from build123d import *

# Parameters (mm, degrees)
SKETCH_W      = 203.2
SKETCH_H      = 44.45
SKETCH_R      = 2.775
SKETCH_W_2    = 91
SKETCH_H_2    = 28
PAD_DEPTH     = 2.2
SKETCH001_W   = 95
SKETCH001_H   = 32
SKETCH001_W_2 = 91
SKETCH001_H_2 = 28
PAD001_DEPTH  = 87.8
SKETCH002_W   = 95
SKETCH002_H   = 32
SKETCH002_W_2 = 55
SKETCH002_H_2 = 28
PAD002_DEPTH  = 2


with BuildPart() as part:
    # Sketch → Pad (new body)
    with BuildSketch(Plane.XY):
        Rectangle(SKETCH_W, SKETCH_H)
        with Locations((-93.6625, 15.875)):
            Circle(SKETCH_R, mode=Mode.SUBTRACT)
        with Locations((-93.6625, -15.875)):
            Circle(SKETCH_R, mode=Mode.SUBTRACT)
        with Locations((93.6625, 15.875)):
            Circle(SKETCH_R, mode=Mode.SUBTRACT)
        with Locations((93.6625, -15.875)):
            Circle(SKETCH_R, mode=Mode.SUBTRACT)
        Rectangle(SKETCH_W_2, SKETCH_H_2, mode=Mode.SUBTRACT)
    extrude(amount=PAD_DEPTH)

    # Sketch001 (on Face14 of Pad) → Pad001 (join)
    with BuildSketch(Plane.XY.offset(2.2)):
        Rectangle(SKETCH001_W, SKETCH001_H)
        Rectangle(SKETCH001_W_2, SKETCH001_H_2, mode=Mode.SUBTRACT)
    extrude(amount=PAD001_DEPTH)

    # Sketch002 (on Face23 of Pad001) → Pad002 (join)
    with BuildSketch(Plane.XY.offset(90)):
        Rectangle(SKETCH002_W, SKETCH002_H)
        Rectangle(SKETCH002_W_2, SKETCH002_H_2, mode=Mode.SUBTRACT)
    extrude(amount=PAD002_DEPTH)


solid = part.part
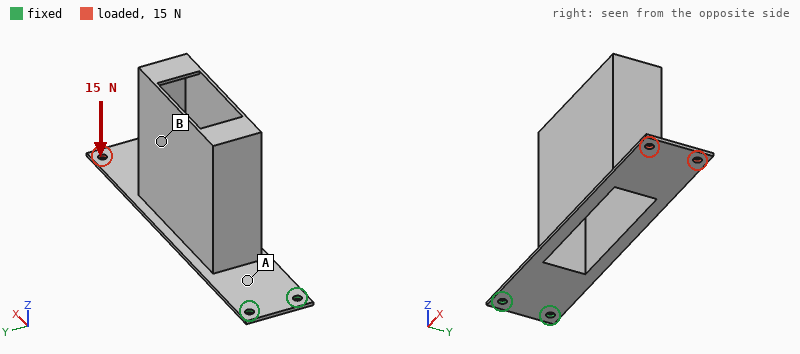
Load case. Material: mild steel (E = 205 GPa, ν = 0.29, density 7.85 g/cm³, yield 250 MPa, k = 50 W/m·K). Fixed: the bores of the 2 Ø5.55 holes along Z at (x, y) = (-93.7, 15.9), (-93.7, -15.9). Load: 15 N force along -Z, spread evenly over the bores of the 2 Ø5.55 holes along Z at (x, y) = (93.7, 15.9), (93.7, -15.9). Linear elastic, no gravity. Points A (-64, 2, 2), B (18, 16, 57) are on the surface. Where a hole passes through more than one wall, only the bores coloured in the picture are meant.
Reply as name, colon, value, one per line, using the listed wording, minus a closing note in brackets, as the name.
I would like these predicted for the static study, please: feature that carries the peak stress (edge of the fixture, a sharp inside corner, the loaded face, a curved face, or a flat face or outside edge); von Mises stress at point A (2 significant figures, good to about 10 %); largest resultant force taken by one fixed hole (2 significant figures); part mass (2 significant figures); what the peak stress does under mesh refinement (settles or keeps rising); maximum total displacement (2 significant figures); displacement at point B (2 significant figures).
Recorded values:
feature that carries the peak stress: edge of the fixture
von Mises stress at point A: 61 MPa
largest resultant force taken by one fixed hole: 7.7 N
part mass: 470 g
what the peak stress does under mesh refinement: keeps rising
maximum total displacement: 2.5 mm
displacement at point B: 1.5 mm
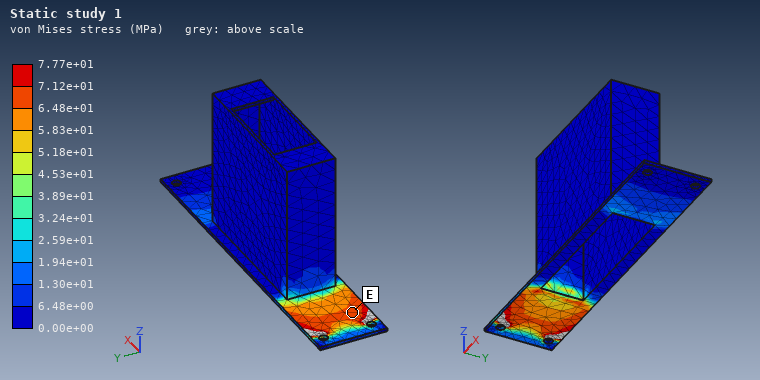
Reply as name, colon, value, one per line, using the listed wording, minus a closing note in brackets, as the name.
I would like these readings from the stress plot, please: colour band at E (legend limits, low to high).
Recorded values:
colour band at E: 6.48e+01 to 7.12e+01 MPa
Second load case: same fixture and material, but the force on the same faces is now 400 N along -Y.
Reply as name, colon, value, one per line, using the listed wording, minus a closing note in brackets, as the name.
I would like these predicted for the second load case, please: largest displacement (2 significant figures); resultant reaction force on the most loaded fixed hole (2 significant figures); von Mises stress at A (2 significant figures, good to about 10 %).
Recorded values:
largest displacement: 0.73 mm
resultant reaction force on the most loaded fixed hole: 2.3 kN
von Mises stress at A: 25 MPa
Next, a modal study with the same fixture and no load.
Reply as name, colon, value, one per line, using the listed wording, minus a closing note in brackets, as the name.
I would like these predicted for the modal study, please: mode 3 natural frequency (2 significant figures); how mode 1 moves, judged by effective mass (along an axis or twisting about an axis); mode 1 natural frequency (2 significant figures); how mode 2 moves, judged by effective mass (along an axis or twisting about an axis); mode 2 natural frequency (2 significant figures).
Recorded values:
mode 3 natural frequency: 350 Hz
how mode 1 moves, judged by effective mass: along Z
mode 1 natural frequency: 32 Hz
how mode 2 moves, judged by effective mass: along Y
mode 2 natural frequency: 97 Hz
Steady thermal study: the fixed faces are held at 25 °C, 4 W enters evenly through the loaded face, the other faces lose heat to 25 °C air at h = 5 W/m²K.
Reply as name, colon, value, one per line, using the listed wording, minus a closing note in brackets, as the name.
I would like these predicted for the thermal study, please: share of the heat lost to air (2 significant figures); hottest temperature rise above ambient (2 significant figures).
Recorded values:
share of the heat lost to air: 87 %
hottest temperature rise above ambient: 60 K
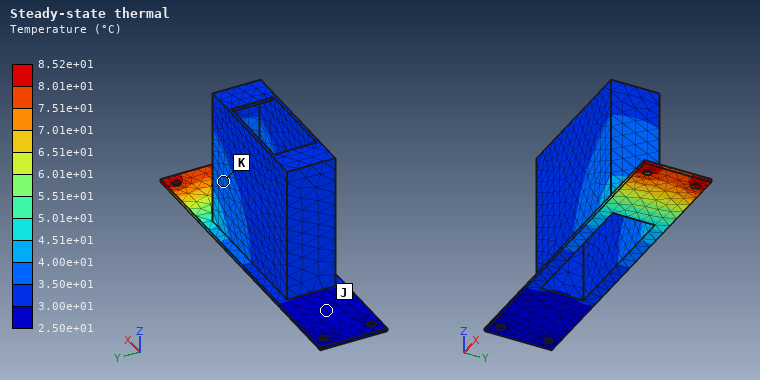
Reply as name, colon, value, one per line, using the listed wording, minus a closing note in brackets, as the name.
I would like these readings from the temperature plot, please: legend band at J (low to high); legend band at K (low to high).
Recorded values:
legend band at J: 2.50e+01 to 3.00e+01 °C
legend band at K: 3.50e+01 to 4.00e+01 °C
